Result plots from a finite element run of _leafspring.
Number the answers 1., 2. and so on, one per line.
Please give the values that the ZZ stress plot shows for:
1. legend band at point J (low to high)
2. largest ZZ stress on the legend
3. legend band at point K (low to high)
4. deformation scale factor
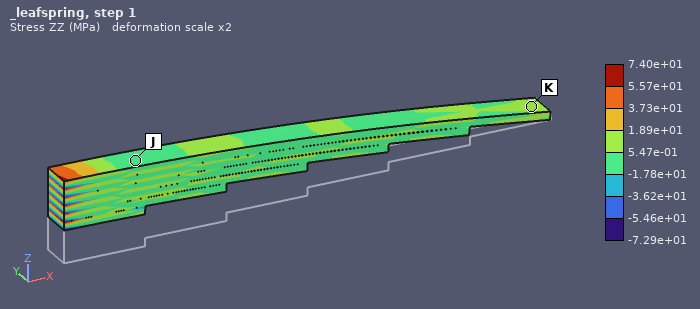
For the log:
1. -1.78e+01 to 5.47e-01 MPa
2. 7.40e+01 MPa
3. 5.47e-01 to 1.89e+01 MPa
4. 2
